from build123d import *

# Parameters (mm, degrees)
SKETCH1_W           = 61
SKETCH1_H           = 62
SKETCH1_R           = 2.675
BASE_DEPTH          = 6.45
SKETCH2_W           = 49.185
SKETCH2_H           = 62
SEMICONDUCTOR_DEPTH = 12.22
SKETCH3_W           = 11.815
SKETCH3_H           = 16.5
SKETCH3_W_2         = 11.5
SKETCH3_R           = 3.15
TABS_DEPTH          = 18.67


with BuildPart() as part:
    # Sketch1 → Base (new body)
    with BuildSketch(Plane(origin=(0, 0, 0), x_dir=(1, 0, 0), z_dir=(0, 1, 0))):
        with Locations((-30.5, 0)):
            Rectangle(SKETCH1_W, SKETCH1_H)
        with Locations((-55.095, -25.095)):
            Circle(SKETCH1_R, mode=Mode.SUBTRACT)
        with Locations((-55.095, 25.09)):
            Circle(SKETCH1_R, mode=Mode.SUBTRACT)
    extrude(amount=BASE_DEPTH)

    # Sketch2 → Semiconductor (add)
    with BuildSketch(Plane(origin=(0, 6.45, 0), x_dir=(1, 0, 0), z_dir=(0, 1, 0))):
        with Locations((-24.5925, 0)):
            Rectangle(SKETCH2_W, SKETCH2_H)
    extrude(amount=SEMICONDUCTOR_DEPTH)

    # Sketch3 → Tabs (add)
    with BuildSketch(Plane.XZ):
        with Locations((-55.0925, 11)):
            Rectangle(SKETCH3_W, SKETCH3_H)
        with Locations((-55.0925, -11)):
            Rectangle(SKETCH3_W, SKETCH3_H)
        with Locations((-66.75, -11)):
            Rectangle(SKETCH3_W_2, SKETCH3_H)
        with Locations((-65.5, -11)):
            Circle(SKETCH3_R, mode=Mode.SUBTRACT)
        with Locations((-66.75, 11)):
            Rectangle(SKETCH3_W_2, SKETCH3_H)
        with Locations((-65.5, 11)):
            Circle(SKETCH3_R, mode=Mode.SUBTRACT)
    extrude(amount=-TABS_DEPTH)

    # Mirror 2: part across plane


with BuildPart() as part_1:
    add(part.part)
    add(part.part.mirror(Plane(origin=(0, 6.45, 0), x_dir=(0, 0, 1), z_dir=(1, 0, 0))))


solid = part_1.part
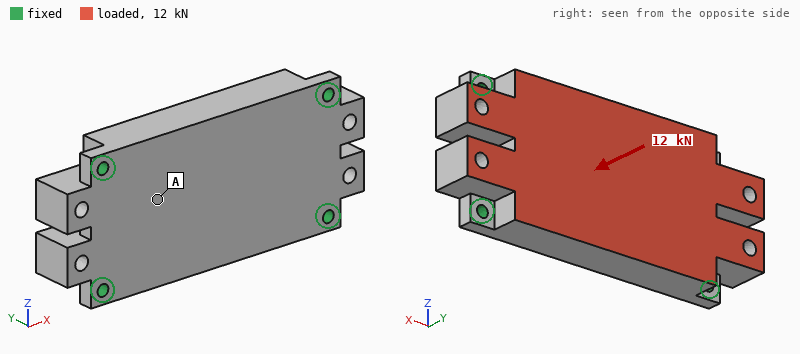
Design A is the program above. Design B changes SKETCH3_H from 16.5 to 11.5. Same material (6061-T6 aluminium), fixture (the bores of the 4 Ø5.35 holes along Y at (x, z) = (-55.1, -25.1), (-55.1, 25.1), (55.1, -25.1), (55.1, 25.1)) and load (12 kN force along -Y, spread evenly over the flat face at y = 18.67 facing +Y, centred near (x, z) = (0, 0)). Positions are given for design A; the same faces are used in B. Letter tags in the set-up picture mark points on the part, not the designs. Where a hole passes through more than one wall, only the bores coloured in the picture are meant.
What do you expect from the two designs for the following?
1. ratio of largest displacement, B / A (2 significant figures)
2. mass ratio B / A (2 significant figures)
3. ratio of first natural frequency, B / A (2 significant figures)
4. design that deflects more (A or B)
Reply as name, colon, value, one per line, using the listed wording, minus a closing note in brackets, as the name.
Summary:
ratio of largest displacement, B / A: 1.1
mass ratio B / A: 0.95
ratio of first natural frequency, B / A: 1.00
design that deflects more: B
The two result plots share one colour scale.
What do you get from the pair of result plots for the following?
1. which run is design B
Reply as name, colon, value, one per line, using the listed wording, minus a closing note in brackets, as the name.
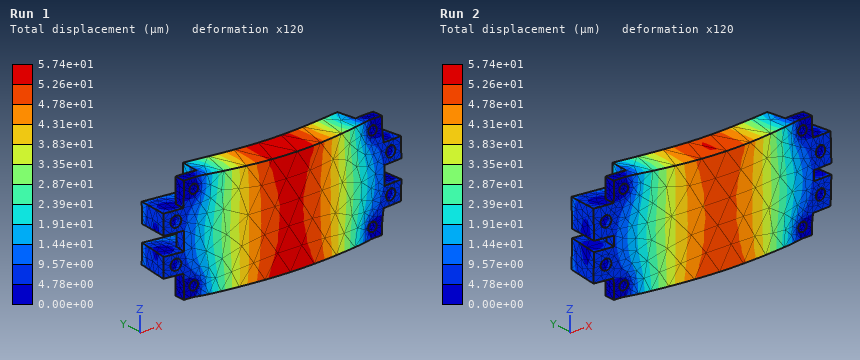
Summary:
which run is design B: Run 1
